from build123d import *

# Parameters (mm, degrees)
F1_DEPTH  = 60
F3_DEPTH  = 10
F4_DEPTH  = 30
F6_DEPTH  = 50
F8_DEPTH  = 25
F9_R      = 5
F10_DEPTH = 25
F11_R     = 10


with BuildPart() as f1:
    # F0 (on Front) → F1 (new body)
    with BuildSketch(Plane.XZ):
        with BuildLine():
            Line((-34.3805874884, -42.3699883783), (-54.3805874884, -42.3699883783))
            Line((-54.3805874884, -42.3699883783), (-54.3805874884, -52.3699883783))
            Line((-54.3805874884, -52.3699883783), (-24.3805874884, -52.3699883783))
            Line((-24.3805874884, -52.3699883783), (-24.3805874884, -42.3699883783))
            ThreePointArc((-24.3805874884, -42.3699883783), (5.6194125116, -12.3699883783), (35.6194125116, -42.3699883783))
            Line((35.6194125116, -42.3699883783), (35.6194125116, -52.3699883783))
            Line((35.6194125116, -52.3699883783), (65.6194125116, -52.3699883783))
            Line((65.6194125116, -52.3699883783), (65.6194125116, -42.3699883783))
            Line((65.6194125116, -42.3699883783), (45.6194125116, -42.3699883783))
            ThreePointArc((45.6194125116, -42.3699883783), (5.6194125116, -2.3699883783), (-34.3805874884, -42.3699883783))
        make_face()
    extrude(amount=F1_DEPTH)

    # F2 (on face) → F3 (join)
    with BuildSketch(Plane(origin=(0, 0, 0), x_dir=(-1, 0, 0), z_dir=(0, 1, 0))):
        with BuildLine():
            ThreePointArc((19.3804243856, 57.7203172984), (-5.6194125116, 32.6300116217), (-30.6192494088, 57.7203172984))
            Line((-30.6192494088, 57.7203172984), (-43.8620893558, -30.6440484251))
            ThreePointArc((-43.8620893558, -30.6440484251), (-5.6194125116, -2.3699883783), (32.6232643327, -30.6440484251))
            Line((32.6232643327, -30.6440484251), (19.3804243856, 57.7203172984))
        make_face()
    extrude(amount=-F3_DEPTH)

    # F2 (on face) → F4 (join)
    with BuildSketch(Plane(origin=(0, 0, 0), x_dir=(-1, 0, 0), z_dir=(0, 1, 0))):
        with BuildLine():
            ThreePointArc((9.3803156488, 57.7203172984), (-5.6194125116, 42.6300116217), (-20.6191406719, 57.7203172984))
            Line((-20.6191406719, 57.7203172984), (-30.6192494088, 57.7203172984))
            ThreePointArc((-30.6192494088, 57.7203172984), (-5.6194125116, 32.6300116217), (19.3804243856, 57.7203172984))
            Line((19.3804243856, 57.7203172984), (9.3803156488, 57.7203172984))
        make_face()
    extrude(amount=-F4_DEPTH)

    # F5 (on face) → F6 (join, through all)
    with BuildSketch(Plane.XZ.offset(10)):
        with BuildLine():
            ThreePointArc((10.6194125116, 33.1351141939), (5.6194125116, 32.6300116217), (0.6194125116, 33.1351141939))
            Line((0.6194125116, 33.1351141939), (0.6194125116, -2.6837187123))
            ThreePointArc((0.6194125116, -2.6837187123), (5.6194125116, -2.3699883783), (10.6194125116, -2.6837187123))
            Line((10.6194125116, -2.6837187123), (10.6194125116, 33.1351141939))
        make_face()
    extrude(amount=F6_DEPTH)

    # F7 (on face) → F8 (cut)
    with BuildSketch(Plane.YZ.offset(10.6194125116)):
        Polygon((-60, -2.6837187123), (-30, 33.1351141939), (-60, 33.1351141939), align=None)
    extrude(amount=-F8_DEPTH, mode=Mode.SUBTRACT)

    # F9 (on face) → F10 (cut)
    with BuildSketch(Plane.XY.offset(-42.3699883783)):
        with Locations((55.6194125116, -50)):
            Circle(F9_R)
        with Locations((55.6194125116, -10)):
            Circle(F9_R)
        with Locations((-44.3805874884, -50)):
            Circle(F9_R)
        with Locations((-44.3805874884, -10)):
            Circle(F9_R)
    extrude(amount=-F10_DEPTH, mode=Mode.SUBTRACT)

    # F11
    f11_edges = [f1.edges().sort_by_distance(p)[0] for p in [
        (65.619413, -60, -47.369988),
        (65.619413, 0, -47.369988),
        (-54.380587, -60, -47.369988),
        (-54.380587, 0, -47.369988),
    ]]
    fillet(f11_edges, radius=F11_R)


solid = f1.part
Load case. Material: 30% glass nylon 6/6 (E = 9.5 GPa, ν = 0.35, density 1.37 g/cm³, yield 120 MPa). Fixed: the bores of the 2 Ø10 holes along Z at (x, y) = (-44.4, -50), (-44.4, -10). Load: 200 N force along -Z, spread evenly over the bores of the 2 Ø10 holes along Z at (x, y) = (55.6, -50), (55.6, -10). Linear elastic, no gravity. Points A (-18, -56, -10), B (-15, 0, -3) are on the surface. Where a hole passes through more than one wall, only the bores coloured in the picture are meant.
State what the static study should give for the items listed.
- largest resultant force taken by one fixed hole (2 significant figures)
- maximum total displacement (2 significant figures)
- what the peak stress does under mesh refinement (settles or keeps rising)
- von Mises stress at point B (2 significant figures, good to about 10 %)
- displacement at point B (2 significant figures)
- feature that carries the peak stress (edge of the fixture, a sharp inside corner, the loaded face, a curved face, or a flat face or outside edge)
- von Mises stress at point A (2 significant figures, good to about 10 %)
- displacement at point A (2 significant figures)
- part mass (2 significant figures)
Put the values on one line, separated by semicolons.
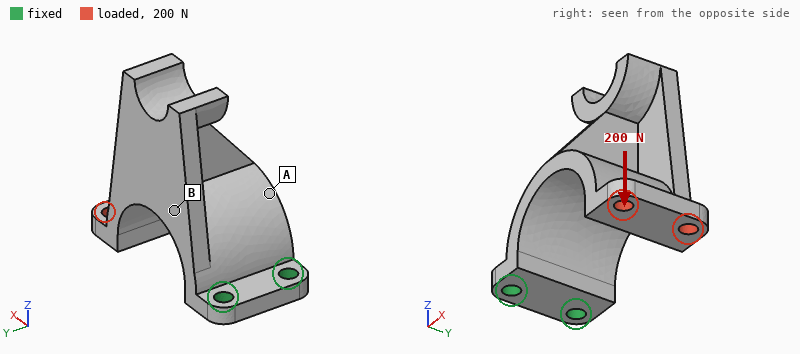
110 N; 1.8 mm; keeps rising; 3.5 MPa; 0.58 mm; edge of the fixture; 9.3 MPa; 0.37 mm; 220 g
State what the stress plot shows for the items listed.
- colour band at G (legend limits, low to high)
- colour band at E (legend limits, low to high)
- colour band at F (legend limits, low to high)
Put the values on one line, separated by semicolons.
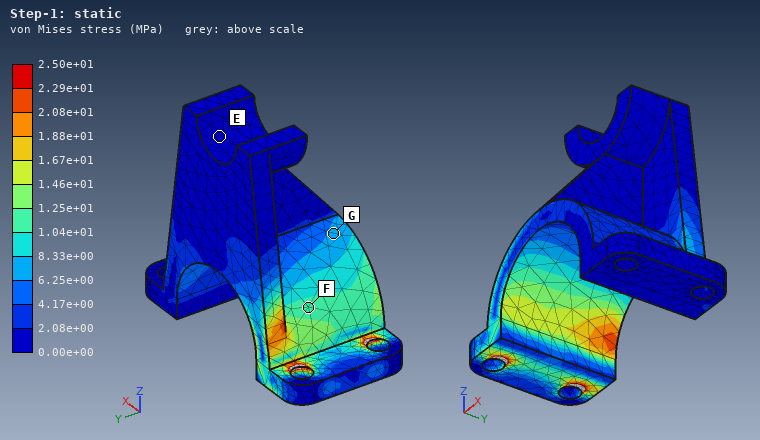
6.25e+00 to 8.33e+00 MPa; 0.00e+00 to 2.08e+00 MPa; 1.04e+01 to 1.25e+01 MPa
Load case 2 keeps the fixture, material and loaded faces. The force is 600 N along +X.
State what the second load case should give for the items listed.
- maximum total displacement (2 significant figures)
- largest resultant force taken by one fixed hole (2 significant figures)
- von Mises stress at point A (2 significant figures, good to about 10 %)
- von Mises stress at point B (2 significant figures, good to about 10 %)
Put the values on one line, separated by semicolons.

1.5 mm; 300 N; 12 MPa; 4.8 MPa
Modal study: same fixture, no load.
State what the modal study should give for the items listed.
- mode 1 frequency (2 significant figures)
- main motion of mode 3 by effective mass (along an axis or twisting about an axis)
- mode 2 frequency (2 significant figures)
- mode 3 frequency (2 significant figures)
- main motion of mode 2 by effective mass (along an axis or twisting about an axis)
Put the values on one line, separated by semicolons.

180 Hz; along Y; 430 Hz; 810 Hz; along Y
